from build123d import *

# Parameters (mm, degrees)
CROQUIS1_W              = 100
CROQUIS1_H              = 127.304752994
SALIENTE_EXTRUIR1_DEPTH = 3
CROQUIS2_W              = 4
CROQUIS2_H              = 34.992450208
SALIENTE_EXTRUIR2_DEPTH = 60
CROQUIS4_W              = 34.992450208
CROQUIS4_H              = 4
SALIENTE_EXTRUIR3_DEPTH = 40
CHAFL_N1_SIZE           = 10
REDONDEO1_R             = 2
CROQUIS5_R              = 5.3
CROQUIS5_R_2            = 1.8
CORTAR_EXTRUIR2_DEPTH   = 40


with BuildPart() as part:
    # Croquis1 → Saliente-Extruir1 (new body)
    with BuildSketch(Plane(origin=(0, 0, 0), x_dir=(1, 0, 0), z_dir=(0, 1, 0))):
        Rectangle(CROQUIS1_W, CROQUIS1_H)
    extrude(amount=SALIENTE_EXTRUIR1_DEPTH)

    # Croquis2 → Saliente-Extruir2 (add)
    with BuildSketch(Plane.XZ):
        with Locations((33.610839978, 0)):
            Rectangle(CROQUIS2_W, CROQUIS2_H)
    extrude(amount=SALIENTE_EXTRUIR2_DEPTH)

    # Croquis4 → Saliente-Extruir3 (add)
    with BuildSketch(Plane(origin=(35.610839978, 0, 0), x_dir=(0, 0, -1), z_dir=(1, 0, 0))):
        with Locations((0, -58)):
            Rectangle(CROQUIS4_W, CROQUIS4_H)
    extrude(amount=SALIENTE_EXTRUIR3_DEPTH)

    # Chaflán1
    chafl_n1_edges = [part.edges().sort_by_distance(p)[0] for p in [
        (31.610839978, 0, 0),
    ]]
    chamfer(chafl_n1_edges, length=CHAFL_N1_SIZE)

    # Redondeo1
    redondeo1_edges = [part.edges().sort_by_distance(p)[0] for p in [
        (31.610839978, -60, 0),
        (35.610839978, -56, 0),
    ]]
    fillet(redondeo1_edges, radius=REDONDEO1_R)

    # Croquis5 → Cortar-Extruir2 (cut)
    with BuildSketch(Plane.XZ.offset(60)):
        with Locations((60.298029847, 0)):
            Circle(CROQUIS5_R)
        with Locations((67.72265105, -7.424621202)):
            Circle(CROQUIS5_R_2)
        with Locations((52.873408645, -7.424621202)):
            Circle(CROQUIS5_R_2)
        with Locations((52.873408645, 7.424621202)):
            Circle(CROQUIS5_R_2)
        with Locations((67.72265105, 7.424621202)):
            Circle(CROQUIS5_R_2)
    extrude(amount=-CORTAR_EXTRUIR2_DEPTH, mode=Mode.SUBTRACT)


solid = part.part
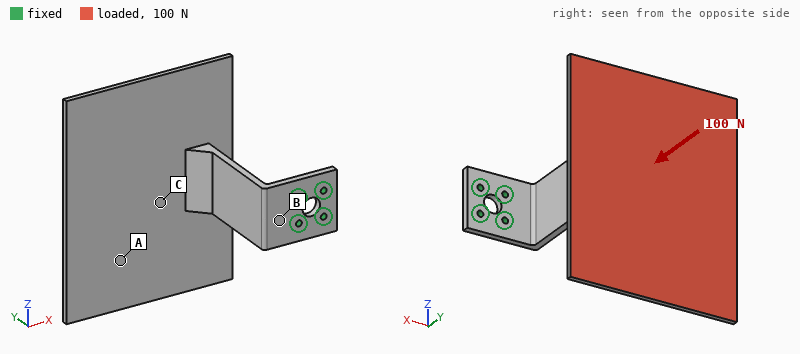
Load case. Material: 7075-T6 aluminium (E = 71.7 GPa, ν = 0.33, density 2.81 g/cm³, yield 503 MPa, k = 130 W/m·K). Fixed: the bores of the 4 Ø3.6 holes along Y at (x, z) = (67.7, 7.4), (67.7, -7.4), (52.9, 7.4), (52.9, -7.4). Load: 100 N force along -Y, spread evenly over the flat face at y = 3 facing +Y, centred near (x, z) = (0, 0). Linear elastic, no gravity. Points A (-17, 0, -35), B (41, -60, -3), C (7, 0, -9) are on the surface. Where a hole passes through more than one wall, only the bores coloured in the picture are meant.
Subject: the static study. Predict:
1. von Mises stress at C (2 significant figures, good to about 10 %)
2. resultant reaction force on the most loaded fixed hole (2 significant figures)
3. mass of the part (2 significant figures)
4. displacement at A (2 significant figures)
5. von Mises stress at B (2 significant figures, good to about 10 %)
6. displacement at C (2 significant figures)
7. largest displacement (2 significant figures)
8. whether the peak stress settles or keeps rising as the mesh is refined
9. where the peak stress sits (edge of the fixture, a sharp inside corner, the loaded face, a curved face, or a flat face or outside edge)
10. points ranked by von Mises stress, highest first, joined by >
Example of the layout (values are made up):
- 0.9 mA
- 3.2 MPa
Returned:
- 11 MPa
- 91 N
- 150 g
- 1.3 mm
- 40 MPa
- 0.89 mm
- 1.9 mm
- keeps rising
- edge of the fixture
- B > C > A
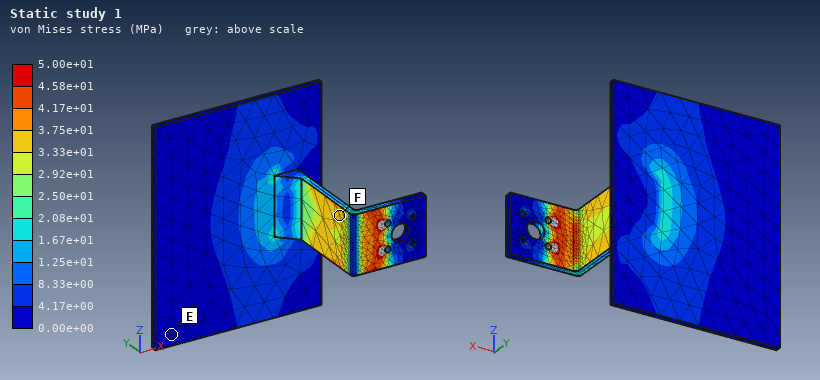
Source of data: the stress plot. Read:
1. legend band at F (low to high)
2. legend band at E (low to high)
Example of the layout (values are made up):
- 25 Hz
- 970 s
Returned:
- 3.33e+01 to 3.75e+01 MPa
- 0.00e+00 to 4.17e+00 MPa
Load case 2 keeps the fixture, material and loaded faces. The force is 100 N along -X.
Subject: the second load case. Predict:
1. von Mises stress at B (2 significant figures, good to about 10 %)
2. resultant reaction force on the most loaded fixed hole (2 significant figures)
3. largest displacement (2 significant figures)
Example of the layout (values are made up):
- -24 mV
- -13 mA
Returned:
- 58 MPa
- 78 N
- 2.0 mm
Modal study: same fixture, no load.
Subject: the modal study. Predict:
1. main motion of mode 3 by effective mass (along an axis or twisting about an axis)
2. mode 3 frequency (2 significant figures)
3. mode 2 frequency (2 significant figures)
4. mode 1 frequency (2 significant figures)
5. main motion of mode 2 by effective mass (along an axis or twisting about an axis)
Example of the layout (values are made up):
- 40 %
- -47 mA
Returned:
- along Z
- 310 Hz
- 190 Hz
- 110 Hz
- along Z
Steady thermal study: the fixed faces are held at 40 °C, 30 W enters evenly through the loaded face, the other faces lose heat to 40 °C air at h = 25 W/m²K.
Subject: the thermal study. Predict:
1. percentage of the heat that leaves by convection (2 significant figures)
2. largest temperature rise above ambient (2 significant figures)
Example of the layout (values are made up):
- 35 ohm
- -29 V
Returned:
- 68 %
- 53 K
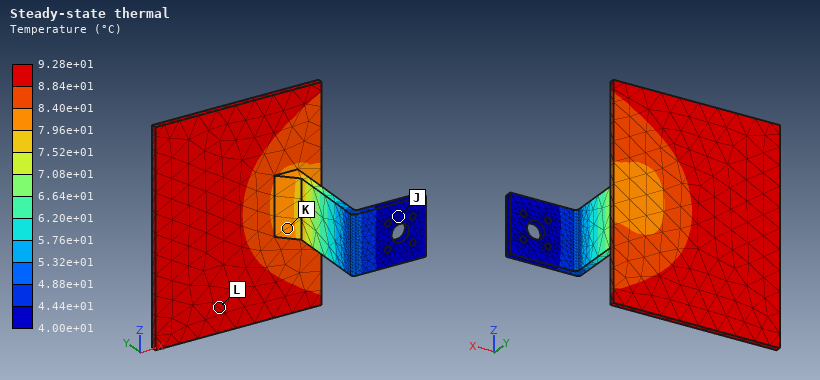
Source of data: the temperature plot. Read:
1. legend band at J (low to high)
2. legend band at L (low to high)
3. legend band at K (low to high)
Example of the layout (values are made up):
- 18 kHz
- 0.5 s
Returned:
- 4.00e+01 to 4.44e+01 °C
- 8.84e+01 to 9.28e+01 °C
- 7.96e+01 to 8.40e+01 °C
